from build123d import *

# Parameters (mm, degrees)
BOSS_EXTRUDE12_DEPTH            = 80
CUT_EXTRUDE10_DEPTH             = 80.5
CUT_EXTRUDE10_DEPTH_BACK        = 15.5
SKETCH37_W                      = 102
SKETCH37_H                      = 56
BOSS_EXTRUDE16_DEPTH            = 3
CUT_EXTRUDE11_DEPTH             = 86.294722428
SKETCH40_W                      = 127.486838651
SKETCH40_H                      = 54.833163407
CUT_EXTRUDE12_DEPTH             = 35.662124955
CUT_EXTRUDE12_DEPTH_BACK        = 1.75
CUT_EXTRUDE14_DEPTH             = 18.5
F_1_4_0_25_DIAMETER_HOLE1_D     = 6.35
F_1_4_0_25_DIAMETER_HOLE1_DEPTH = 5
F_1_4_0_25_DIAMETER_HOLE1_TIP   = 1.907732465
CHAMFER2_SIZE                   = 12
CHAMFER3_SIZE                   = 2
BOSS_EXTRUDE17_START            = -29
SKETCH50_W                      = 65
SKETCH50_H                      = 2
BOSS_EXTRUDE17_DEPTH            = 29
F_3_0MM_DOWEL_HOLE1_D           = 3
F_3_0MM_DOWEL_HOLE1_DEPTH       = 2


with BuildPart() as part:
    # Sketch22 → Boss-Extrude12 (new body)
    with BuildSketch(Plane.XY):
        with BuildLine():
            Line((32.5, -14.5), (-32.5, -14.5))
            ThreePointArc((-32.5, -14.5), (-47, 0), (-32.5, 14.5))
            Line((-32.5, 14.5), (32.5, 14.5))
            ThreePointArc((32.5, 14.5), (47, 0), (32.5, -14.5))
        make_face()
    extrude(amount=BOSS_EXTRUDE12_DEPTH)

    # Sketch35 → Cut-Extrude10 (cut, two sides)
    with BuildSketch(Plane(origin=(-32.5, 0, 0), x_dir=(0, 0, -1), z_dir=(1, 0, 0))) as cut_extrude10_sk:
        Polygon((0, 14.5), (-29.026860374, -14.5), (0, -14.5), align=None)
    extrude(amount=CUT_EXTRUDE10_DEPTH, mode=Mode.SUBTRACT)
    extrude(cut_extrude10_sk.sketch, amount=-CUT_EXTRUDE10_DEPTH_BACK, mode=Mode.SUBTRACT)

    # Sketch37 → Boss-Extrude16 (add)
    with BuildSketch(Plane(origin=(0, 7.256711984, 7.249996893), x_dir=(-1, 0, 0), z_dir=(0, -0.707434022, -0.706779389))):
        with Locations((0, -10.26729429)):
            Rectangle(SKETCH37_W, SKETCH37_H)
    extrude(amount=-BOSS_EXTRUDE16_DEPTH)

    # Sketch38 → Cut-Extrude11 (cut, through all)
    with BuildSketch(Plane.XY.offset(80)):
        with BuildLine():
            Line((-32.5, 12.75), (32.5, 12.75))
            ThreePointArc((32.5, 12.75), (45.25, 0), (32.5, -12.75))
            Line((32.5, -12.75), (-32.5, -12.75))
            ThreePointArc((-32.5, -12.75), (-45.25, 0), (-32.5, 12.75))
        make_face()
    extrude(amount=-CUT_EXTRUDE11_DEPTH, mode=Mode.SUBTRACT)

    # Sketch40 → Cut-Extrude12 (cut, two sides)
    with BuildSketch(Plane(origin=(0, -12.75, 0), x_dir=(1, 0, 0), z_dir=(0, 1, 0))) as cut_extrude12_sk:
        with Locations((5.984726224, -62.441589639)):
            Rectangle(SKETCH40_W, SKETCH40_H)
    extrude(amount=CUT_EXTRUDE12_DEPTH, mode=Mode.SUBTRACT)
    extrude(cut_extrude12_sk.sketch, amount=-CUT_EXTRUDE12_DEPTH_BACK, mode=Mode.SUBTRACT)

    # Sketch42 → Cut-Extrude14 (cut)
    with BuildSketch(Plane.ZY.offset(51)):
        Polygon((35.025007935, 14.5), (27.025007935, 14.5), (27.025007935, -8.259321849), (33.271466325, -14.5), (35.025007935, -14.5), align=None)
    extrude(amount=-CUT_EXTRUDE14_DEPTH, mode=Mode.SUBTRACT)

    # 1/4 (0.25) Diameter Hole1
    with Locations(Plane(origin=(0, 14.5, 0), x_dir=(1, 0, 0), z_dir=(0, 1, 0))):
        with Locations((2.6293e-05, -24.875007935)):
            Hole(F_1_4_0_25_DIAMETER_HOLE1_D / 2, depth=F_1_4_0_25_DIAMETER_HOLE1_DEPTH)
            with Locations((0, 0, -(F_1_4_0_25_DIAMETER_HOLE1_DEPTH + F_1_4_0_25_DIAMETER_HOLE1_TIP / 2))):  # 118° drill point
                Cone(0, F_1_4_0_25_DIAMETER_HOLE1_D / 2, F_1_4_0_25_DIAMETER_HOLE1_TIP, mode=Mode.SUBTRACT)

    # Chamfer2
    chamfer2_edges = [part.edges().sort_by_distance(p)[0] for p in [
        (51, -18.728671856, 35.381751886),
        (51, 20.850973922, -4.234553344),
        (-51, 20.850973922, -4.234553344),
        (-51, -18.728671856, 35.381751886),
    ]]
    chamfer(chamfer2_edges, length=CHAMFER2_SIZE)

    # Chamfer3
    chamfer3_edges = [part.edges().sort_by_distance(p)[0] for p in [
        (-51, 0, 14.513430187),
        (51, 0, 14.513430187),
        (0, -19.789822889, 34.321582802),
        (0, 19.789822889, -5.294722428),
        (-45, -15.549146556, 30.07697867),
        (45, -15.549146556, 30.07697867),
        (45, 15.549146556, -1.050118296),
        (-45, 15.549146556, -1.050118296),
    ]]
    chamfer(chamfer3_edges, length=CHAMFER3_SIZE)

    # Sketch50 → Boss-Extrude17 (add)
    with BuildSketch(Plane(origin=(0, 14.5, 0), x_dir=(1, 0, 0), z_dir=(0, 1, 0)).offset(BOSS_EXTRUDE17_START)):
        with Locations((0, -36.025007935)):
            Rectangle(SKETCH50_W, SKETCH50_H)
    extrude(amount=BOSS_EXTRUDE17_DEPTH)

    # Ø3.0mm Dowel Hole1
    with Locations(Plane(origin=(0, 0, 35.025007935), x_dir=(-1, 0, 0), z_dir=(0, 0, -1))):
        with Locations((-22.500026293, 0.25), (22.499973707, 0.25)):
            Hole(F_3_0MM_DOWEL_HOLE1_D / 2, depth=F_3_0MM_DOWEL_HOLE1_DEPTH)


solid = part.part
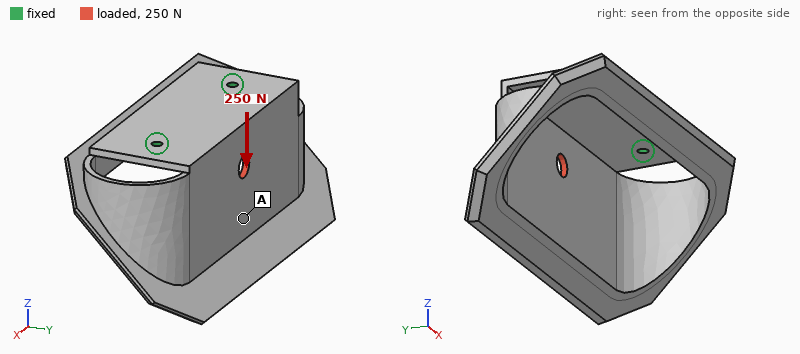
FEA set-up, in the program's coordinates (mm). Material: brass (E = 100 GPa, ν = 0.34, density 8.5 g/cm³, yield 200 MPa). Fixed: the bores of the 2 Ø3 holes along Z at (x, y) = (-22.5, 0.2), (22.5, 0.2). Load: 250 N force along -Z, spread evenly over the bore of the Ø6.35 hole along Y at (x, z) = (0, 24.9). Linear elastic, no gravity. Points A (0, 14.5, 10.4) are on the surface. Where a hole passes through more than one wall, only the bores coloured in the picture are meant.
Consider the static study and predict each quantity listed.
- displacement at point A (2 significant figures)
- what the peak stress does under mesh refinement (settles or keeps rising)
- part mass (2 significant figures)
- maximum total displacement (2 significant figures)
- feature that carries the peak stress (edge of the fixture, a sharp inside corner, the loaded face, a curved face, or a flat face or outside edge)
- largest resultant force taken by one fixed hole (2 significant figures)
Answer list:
0.12 mm
keeps rising
130 g
0.17 mm
edge of the fixture
130 N
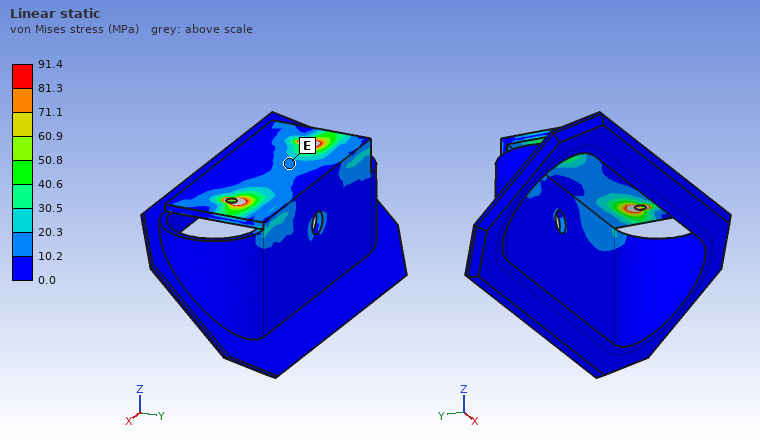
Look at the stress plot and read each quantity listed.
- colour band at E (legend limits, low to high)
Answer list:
10.2 to 20.3 MPa
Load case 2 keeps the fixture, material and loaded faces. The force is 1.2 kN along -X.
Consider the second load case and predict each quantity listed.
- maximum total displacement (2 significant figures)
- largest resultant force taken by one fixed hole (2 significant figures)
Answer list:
0.16 mm
750 N
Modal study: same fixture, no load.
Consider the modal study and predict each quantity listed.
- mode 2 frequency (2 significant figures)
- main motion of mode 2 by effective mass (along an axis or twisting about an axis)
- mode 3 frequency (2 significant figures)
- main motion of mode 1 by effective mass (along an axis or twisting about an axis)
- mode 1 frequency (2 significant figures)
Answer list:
1000 Hz
along X
1400 Hz
along Y
510 Hz
